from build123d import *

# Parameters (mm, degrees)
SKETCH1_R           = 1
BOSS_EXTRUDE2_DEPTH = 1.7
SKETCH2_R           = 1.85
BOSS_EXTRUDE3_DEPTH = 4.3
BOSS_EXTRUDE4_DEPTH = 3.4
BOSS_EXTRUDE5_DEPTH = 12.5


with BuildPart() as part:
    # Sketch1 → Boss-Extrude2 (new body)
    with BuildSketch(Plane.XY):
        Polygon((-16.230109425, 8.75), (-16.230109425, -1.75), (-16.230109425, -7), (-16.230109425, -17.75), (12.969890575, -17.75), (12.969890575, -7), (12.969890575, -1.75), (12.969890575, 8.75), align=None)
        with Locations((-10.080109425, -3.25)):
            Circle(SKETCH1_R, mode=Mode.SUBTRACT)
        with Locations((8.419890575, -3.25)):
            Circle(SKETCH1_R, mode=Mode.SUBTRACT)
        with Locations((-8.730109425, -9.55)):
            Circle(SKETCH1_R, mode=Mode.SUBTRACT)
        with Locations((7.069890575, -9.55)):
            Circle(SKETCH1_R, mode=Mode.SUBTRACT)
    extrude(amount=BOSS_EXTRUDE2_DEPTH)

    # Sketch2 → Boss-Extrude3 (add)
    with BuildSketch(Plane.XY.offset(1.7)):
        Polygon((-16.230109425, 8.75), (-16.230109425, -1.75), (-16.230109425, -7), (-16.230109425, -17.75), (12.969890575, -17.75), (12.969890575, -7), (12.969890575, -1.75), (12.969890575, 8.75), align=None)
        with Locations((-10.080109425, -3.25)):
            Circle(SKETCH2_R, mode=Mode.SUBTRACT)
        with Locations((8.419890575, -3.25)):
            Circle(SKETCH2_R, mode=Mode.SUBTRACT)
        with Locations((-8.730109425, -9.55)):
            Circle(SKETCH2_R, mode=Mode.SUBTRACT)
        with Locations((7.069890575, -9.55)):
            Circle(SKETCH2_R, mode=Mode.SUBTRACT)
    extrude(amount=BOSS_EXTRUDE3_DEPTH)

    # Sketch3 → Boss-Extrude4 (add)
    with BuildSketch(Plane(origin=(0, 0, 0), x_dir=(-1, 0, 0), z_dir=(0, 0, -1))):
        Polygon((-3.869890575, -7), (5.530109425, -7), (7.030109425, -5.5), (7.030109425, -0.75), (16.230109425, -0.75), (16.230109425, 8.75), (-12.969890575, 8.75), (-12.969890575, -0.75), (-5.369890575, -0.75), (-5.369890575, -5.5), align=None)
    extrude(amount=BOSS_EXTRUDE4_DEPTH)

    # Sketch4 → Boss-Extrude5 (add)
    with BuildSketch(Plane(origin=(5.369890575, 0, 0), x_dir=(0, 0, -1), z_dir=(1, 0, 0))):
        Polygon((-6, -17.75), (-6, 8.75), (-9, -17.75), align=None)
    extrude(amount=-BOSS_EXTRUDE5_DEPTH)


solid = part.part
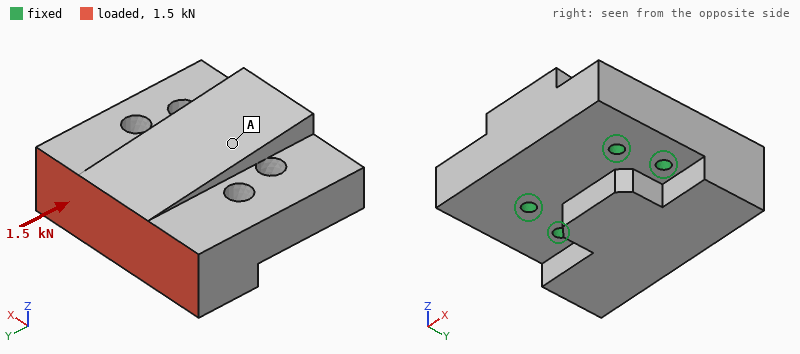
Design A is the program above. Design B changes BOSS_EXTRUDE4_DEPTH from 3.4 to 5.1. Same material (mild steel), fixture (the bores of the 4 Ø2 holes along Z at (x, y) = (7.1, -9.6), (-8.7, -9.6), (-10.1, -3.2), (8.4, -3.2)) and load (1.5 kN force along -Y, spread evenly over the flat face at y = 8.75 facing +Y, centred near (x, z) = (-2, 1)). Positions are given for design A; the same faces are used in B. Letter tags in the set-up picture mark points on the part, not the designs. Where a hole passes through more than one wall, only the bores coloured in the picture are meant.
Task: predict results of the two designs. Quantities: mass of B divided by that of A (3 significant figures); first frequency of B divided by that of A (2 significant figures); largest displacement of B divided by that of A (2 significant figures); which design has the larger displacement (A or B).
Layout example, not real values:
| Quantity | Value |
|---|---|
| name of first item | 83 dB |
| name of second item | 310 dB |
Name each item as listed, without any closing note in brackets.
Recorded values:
| Quantity | Value |
|---|---|
| mass of B divided by that of A | 1.10 |
| first frequency of B divided by that of A | 0.93 |
| largest displacement of B divided by that of A | 2.0 |
| which design has the larger displacement | B |
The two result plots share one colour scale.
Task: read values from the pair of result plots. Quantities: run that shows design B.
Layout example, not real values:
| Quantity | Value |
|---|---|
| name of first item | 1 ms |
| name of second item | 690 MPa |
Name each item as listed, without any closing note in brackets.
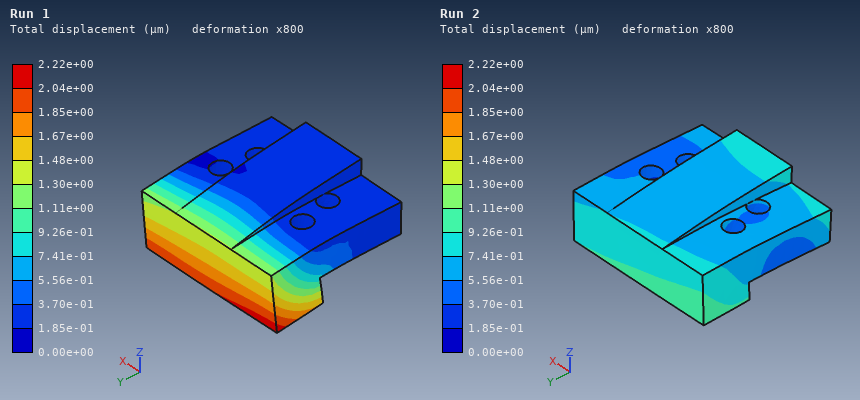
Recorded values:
| Quantity | Value |
|---|---|
| run that shows design B | Run 1 |
